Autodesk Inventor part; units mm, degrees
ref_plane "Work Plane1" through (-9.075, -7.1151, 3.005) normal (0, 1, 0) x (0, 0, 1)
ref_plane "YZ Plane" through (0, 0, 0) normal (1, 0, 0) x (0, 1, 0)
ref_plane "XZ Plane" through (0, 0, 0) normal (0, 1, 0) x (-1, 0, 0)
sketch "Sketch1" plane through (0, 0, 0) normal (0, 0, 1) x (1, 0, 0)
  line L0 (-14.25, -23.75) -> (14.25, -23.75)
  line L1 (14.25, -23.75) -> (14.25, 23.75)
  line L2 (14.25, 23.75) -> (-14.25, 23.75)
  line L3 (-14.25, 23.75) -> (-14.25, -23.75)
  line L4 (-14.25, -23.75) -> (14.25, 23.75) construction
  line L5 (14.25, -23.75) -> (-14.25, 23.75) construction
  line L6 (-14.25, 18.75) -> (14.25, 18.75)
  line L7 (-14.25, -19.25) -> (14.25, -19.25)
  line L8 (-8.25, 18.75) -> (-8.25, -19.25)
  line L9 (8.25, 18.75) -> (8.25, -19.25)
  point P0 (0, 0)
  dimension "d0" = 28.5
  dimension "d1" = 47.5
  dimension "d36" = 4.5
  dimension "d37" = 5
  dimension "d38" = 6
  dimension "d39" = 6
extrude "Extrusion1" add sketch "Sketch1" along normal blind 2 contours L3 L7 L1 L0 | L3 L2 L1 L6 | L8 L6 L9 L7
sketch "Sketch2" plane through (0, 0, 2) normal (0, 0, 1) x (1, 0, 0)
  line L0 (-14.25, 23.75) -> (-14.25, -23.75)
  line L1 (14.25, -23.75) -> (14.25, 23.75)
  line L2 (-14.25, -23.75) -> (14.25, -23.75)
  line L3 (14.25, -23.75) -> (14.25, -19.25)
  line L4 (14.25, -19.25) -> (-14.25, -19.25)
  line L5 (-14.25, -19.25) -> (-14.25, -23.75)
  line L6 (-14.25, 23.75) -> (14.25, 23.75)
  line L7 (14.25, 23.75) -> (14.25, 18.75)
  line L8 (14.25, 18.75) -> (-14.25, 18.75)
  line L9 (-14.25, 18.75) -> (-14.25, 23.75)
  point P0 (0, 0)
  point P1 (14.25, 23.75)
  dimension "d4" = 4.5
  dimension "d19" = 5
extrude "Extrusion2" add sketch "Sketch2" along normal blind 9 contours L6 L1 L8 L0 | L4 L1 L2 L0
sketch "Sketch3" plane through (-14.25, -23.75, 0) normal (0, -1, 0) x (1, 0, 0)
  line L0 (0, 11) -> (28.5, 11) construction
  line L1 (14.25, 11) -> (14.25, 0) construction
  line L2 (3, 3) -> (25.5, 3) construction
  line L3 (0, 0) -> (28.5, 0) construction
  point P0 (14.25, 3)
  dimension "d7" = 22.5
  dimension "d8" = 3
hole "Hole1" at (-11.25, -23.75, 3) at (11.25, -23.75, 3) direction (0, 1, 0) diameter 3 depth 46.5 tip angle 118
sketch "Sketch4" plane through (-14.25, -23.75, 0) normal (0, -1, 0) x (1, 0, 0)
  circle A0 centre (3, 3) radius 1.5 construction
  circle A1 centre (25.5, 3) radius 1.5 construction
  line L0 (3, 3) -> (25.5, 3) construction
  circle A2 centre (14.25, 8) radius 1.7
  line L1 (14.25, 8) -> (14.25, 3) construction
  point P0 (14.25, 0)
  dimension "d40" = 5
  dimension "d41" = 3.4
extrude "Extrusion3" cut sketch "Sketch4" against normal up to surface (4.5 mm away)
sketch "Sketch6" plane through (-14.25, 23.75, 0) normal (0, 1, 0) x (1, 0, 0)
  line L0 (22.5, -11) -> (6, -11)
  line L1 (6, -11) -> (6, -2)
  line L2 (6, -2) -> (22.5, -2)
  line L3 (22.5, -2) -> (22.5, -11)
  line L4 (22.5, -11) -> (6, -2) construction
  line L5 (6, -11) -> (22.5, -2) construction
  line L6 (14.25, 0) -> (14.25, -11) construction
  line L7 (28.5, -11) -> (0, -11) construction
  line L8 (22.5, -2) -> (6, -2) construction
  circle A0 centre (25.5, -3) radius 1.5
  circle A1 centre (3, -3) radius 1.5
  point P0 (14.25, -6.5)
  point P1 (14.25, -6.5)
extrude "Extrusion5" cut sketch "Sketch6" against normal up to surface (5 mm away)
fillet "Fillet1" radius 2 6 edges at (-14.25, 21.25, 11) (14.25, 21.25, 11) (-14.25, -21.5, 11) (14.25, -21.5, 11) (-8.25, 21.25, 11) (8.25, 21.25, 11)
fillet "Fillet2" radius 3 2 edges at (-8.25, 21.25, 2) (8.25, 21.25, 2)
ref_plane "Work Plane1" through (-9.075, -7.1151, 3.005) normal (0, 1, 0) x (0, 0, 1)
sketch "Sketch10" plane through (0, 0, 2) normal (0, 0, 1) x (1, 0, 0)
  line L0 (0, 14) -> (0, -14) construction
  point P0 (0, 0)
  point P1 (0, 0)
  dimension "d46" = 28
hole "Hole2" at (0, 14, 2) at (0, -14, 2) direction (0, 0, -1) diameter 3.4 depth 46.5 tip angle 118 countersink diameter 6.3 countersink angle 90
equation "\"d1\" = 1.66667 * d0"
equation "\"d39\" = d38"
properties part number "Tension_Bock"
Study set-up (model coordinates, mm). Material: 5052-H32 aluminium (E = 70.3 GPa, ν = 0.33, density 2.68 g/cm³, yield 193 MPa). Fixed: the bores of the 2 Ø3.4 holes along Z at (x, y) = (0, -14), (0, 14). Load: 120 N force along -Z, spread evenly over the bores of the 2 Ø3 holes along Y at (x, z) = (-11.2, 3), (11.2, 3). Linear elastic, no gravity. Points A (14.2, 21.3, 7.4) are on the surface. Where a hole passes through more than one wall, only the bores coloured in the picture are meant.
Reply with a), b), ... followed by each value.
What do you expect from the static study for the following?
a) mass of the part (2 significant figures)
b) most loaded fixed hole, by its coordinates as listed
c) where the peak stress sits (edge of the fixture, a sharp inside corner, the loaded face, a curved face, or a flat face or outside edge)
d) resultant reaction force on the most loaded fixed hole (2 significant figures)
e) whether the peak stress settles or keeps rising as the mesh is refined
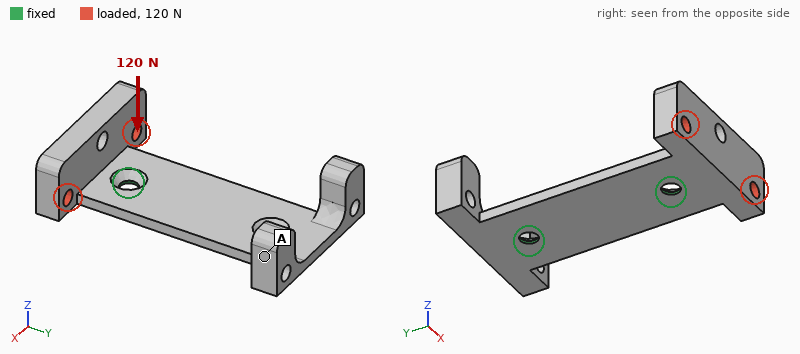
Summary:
a) 8.7 g
b) (0, -14)
c) edge of the fixture
d) 180 N
e) keeps rising
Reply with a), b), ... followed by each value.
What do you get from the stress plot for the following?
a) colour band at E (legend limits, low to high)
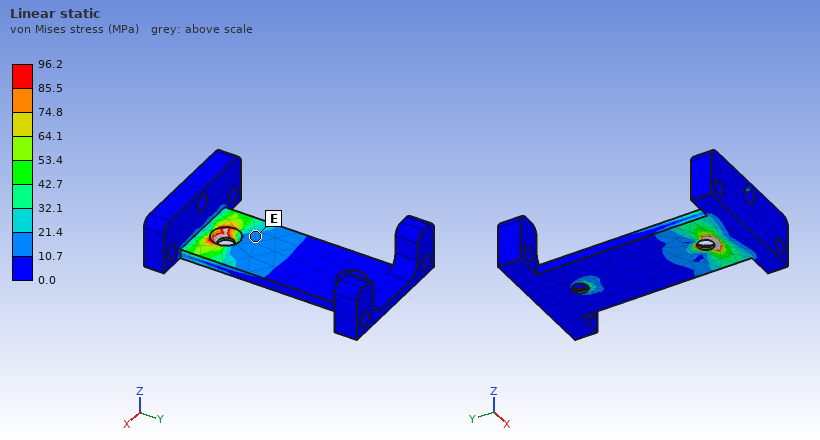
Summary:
a) 10.7 to 21.4 MPa
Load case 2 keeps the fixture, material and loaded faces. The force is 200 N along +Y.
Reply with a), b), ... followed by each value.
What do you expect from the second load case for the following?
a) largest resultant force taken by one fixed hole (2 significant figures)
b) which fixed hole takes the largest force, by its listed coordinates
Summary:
a) 110 N
b) (0, 14)
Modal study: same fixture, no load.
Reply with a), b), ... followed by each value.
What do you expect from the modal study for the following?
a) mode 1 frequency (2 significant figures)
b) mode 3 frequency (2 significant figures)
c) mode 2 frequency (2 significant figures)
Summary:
a) 2800 Hz
b) 3200 Hz
c) 3100 Hz
